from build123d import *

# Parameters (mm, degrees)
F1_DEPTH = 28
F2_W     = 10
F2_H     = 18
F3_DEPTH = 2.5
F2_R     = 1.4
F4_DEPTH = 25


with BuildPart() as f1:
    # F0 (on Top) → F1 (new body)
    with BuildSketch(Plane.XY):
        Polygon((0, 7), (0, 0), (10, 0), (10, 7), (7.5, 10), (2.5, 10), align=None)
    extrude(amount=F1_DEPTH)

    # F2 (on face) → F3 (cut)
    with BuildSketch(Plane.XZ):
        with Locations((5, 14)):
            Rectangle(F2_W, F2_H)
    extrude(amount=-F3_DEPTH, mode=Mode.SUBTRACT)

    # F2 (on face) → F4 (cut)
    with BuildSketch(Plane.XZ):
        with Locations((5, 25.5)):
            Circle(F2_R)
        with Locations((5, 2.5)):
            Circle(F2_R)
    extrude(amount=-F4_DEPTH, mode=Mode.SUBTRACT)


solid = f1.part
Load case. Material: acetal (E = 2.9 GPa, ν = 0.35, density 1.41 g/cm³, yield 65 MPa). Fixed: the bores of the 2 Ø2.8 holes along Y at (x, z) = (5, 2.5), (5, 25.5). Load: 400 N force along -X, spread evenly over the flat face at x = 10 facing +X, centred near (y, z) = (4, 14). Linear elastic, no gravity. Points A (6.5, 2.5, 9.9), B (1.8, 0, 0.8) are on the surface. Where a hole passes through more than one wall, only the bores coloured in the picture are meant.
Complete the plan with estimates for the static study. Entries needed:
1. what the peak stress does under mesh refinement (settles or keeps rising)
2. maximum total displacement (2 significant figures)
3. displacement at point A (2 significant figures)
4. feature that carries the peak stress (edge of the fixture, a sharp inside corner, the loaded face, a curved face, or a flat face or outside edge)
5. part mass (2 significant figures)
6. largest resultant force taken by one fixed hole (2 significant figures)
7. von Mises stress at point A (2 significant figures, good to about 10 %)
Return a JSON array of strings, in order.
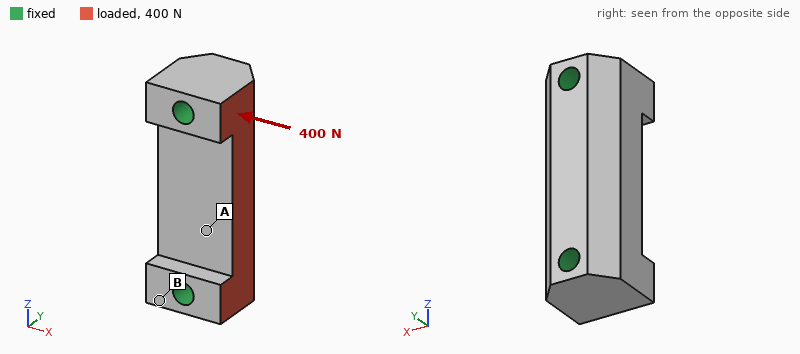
["keeps rising", "31 µm", "23 µm", "edge of the fixture", "2.8 g", "200 N", "3.5 MPa"]
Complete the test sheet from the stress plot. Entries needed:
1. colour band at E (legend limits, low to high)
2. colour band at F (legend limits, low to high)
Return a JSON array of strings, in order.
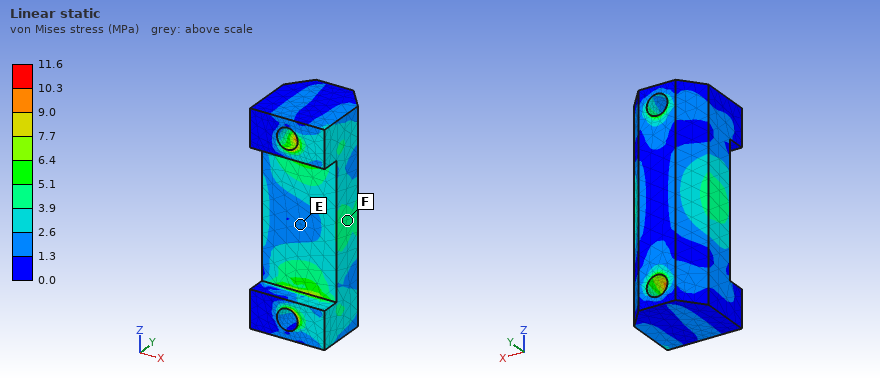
["1.3 to 2.6 MPa", "3.9 to 5.1 MPa"]
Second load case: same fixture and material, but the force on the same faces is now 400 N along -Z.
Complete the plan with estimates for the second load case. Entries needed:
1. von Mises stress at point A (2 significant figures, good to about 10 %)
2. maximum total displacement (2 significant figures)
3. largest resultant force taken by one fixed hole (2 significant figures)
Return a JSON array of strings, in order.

["3.3 MPa", "25 µm", "210 N"]
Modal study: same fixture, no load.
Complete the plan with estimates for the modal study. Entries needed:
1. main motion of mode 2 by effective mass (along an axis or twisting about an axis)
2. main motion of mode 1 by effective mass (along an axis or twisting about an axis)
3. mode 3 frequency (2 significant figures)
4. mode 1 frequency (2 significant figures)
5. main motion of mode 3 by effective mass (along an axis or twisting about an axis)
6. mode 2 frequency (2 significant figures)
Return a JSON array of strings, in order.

["along Y", "along X", "19 kHz", "13 kHz", "twisting about Z", "14 kHz"]
